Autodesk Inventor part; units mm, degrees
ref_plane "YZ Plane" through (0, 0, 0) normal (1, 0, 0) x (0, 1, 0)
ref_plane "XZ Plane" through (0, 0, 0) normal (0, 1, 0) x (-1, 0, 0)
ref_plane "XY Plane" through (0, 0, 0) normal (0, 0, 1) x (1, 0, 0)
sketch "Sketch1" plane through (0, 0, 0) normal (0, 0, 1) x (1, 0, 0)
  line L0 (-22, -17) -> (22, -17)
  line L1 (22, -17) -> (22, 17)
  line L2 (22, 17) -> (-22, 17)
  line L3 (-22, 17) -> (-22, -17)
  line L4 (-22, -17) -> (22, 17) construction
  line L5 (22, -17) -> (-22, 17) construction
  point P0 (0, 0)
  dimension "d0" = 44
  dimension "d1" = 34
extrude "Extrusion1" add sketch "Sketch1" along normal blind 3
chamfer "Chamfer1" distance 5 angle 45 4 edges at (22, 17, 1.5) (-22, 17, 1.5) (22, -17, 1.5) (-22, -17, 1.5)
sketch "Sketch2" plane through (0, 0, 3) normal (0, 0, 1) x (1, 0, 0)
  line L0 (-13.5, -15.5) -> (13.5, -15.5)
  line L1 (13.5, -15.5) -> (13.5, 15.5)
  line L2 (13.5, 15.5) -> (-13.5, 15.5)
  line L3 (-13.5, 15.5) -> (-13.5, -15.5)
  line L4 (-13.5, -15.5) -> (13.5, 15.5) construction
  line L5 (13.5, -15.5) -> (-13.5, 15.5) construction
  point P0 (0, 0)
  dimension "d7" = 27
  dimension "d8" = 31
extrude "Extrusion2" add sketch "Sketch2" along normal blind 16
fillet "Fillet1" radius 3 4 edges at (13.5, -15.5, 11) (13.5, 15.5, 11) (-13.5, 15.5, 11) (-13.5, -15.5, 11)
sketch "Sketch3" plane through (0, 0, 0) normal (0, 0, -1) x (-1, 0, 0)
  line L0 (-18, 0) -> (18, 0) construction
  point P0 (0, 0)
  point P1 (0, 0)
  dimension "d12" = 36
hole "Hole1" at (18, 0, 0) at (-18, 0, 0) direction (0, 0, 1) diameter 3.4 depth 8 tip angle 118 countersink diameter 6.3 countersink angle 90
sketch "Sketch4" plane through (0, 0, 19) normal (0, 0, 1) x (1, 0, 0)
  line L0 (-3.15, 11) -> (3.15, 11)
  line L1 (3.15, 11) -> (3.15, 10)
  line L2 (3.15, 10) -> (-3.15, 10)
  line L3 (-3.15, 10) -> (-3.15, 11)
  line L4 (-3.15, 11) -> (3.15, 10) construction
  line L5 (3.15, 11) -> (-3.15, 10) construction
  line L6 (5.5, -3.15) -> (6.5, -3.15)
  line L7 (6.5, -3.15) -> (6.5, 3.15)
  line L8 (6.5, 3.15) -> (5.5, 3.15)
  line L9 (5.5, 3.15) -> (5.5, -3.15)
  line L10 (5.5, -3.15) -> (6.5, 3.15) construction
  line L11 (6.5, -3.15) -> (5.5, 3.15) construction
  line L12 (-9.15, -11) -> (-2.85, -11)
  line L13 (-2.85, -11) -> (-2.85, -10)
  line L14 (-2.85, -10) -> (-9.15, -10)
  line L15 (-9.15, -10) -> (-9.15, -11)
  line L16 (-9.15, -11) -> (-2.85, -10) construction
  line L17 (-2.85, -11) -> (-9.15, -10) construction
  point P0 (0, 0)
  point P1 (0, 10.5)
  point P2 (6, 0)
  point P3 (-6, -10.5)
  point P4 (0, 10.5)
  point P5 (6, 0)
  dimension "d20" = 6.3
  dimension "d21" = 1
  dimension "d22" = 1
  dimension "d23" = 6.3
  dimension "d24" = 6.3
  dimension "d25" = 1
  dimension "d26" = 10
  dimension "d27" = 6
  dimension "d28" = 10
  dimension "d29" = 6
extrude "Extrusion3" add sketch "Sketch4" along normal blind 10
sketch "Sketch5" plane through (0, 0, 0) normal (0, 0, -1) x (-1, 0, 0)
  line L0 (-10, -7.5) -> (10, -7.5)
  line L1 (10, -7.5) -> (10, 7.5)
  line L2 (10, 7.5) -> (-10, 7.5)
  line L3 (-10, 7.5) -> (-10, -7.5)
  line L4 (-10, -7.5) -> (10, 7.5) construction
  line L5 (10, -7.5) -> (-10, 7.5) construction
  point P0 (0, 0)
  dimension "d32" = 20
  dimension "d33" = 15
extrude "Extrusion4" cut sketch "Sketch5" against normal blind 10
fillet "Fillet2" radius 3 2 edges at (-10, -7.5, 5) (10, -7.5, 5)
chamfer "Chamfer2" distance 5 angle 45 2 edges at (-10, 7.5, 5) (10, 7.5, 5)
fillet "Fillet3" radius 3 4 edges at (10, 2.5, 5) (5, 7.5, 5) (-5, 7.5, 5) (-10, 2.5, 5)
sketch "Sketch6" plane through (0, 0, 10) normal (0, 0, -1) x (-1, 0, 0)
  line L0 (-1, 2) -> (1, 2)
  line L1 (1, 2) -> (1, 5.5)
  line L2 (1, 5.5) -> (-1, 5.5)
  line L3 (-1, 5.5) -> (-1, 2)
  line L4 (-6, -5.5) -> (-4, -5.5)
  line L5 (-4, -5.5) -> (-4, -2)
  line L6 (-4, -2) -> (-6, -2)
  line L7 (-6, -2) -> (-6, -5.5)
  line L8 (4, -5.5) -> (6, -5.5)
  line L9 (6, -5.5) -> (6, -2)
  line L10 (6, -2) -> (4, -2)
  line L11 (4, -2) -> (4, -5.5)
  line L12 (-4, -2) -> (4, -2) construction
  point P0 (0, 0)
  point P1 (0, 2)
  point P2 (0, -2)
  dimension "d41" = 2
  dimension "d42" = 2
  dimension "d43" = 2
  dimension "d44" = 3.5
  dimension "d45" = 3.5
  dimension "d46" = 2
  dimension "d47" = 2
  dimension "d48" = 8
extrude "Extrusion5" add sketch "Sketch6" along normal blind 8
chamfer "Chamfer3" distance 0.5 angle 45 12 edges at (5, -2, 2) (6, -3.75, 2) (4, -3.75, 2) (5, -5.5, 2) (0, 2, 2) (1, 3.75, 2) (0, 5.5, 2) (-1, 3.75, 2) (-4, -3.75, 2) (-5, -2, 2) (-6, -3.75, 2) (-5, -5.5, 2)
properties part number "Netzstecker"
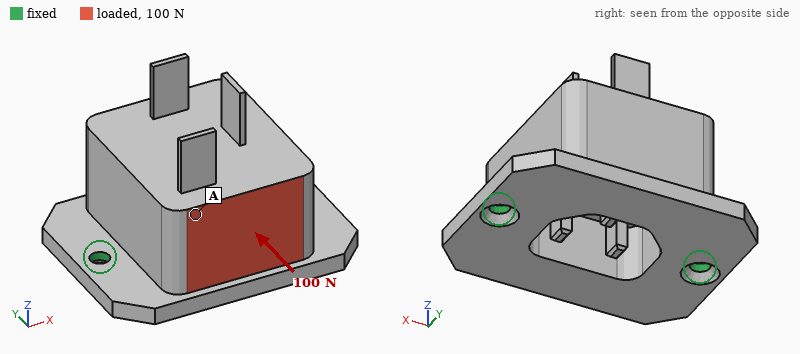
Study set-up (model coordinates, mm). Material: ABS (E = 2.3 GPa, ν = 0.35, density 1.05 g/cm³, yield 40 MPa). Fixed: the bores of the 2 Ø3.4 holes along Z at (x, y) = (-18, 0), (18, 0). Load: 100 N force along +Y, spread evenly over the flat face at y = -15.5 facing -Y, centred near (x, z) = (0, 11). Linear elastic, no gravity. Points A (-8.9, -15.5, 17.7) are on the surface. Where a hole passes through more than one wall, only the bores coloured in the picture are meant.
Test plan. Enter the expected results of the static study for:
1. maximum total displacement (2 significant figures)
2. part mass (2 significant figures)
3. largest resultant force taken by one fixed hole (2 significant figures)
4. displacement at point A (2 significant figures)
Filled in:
0.72 mm
16 g
50 N
0.55 mm
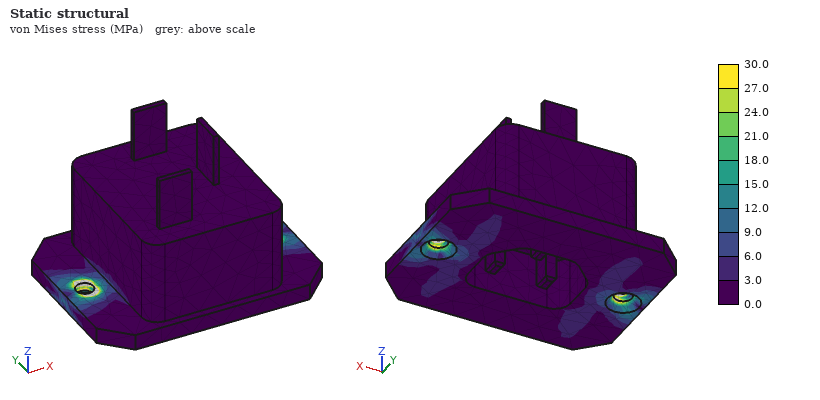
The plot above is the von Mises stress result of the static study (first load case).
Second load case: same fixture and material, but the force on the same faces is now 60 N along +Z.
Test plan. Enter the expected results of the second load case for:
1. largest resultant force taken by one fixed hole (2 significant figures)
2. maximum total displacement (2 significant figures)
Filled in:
33 N
0.75 mm
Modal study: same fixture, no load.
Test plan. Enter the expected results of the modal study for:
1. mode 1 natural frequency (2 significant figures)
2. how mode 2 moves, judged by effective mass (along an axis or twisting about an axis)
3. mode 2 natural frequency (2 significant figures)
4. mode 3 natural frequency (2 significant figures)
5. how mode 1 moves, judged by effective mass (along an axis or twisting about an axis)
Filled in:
560 Hz
along Z
2200 Hz
2300 Hz
along Y
